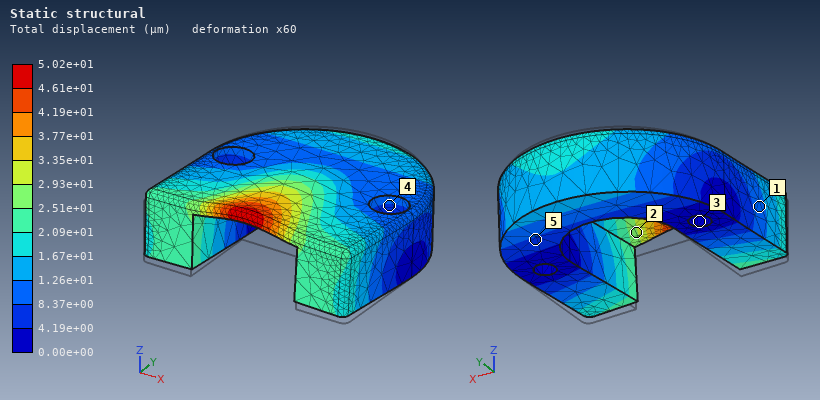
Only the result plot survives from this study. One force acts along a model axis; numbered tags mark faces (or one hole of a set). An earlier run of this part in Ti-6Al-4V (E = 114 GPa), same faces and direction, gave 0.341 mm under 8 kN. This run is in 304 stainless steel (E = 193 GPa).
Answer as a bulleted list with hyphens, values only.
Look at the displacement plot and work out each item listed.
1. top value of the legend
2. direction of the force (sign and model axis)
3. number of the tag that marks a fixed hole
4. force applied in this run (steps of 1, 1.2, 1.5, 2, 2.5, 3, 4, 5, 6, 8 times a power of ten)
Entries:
- 5.02e+01 µm
- +Z
- 3
- 2 kN
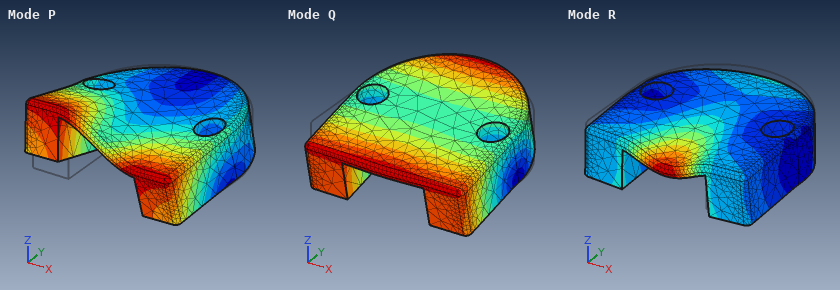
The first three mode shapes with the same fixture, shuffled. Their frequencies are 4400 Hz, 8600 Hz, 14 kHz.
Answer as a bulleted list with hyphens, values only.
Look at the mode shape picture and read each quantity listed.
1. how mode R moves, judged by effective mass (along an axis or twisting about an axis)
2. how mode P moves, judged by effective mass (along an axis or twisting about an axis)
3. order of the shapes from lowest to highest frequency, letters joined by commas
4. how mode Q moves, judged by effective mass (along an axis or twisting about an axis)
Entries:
- along Z
- along X
- Q, P, R
- along Y
